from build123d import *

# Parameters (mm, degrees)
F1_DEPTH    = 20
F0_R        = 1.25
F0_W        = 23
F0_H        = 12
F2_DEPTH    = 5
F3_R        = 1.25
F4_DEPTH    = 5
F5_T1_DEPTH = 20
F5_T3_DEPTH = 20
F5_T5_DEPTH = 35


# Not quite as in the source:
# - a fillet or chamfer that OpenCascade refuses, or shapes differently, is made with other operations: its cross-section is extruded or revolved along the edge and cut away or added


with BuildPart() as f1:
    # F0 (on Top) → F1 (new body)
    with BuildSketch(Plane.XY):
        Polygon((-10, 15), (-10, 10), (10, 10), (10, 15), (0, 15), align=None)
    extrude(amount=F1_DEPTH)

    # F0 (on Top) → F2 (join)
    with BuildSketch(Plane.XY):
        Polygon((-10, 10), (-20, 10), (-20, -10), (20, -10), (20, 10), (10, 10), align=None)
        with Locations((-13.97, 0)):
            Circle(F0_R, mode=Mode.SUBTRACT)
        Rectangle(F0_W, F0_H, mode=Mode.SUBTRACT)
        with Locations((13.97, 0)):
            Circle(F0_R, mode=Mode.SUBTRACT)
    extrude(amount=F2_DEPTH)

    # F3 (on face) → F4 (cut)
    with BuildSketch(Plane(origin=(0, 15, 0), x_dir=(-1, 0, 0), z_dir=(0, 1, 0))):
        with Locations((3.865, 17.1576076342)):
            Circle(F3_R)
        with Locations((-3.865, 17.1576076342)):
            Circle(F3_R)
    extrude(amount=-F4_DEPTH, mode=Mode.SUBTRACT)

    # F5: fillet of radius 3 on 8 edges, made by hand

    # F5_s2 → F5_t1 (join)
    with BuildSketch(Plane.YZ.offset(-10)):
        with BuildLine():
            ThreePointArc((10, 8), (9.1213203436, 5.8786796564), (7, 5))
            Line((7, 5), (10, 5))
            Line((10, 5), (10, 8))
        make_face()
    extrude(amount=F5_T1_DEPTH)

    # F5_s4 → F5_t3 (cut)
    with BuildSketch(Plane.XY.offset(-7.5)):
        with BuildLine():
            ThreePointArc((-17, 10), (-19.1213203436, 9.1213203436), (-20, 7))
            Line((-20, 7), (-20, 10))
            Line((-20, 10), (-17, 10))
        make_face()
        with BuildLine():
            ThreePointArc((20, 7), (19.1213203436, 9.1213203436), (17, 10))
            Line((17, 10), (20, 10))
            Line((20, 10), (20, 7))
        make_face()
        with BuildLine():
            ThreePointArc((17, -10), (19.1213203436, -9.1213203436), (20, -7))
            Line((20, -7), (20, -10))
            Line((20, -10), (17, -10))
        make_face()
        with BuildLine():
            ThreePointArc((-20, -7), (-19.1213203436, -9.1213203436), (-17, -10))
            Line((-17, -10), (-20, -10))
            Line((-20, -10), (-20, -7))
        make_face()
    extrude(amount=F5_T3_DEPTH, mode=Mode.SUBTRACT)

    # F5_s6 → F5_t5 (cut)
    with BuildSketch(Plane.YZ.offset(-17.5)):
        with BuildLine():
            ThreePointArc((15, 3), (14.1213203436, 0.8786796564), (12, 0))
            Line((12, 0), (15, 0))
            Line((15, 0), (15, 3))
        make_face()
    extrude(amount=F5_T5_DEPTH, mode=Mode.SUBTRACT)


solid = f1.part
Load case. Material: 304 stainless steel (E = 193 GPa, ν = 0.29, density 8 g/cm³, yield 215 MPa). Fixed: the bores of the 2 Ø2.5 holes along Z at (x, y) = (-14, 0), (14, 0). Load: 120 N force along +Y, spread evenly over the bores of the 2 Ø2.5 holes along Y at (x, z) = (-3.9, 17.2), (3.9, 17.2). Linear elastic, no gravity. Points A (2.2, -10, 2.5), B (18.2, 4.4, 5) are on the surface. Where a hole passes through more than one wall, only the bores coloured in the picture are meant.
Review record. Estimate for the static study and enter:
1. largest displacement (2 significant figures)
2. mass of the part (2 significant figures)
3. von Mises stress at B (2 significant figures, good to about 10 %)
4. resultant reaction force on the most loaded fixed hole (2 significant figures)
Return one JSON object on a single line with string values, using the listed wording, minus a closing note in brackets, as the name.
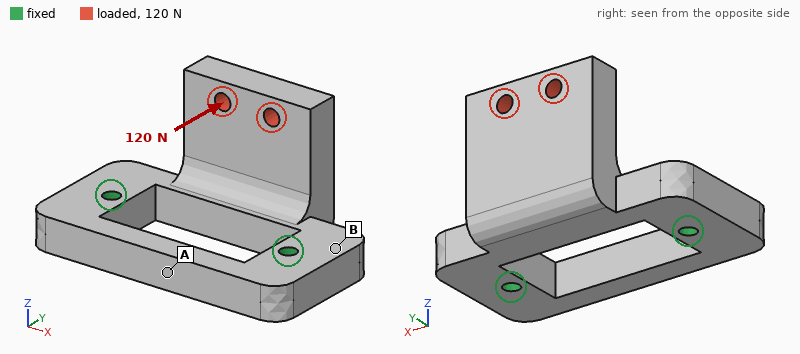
{"largest displacement": "29 µm", "mass of the part": "36 g", "von Mises stress at B": "15 MPa", "resultant reaction force on the most loaded fixed hole": "72 N"}
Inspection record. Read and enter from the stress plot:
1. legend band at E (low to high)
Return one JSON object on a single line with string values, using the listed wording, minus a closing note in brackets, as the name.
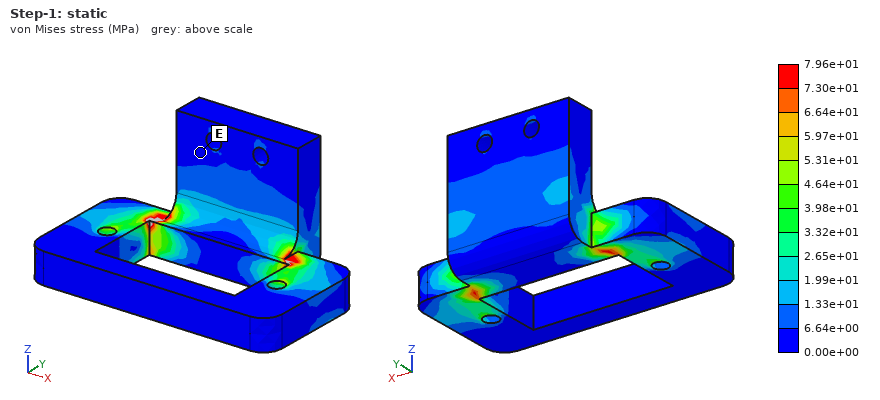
{"legend band at E": "0.00e+00 to 6.64e+00 MPa"}
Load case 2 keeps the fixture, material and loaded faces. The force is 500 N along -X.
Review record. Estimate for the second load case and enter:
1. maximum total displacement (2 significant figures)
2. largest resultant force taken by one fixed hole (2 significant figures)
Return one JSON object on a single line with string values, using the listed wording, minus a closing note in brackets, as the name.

{"maximum total displacement": "16 µm", "largest resultant force taken by one fixed hole": "390 N"}
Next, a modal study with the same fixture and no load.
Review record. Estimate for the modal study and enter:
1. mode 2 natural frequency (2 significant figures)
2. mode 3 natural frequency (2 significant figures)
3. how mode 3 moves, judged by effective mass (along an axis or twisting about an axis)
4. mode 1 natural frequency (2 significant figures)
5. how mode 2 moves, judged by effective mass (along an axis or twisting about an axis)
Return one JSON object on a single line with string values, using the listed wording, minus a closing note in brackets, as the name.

{"mode 2 natural frequency": "11 kHz", "mode 3 natural frequency": "11 kHz", "how mode 3 moves, judged by effective mass": "along Z", "mode 1 natural frequency": "4000 Hz", "how mode 2 moves, judged by effective mass": "along X"}
